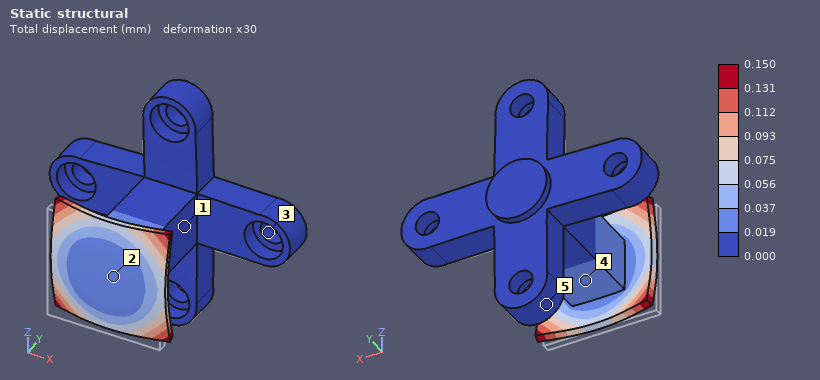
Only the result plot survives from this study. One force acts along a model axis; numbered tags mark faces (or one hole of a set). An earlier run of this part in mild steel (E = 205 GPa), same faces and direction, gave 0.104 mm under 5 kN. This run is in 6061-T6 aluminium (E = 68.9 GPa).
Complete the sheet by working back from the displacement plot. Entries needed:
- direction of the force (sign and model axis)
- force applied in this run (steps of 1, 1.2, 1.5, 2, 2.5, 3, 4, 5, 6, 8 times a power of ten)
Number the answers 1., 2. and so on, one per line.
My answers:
1. +Y
2. 2.5 kN
